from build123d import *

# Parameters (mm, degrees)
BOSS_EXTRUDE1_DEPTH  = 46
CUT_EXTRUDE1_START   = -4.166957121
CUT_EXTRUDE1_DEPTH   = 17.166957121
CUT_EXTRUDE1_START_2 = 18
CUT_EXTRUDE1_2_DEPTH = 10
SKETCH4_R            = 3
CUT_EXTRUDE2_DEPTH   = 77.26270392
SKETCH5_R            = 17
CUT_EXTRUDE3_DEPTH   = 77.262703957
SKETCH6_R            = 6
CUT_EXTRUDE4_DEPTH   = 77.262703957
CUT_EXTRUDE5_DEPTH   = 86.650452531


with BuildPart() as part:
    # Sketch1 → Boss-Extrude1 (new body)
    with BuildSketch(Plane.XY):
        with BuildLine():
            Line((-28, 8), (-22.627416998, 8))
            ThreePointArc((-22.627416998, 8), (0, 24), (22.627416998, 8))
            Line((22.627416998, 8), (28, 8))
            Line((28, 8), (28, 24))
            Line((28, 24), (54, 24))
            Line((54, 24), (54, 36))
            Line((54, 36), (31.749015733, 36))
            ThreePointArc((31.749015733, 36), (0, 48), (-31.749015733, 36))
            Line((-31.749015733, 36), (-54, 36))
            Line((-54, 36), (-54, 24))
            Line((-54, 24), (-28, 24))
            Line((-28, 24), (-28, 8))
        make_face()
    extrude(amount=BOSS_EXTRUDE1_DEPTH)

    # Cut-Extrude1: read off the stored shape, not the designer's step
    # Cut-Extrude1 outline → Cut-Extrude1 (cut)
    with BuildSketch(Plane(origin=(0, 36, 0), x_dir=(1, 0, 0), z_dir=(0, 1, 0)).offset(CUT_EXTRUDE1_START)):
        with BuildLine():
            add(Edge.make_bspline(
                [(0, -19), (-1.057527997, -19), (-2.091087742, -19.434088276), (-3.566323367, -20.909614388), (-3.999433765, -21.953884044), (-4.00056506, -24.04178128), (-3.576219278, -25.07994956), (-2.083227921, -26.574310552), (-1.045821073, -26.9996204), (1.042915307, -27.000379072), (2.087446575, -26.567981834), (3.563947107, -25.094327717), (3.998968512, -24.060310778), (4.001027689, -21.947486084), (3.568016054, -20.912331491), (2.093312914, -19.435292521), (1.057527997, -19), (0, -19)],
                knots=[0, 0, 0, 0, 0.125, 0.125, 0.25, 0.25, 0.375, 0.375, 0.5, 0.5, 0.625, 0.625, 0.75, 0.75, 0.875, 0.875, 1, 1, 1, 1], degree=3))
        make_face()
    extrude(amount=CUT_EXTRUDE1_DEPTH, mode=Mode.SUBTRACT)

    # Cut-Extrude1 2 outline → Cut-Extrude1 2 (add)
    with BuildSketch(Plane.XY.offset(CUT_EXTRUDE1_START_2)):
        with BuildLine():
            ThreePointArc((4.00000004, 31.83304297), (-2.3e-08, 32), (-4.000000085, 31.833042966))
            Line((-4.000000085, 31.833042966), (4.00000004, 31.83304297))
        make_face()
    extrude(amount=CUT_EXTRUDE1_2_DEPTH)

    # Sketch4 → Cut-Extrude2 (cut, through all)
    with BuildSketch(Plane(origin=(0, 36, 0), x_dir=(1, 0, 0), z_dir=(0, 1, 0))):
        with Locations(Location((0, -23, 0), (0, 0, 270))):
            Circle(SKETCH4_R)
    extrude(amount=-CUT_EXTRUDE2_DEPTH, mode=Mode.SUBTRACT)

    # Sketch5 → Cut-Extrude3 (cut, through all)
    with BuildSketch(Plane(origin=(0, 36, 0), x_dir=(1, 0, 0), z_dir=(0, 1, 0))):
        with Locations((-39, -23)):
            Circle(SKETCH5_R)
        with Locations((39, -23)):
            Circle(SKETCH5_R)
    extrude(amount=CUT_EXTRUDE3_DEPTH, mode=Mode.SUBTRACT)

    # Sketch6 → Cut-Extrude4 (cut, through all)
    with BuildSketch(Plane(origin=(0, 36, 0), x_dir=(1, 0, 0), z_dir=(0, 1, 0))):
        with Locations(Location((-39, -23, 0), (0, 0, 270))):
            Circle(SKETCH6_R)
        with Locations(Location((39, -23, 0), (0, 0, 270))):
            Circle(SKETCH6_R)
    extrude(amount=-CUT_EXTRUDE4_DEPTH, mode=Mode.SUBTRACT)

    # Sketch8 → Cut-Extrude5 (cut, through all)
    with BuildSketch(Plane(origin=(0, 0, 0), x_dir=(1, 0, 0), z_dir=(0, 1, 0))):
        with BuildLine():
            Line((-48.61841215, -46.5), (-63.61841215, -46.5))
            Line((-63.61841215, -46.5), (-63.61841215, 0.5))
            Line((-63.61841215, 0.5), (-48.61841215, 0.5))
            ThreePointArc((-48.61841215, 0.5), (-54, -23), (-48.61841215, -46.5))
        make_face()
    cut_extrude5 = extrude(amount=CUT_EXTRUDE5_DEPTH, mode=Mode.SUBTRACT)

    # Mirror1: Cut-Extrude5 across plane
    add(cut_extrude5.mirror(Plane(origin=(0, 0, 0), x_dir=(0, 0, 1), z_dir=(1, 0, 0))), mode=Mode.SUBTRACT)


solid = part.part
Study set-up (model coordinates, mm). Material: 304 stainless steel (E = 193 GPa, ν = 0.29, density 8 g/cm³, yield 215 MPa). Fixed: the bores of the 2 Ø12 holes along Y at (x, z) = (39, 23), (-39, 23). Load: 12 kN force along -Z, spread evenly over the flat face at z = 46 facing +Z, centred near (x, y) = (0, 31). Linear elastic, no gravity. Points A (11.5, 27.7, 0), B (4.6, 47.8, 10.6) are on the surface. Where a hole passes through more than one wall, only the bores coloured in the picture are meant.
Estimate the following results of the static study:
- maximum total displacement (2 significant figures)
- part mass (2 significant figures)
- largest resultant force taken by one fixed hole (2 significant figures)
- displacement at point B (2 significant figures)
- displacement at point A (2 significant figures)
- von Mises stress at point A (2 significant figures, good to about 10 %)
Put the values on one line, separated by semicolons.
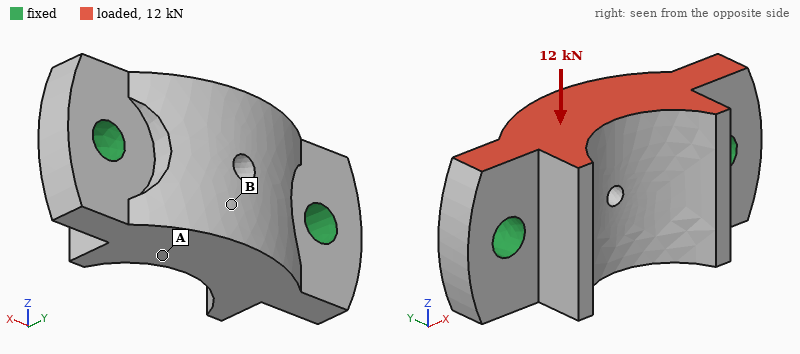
5.5 µm; 750 g; 6.0 kN; 4.4 µm; 3.1 µm; 12 MPa
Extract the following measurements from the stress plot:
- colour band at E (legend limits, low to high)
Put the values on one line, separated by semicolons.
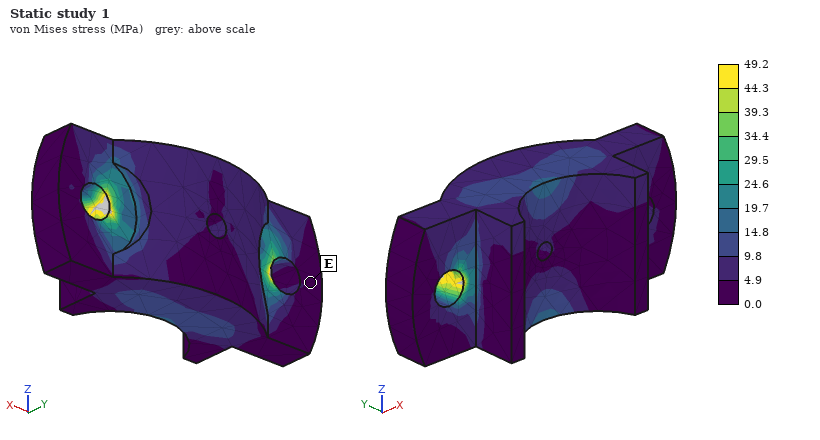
0.0 to 4.9 MPa
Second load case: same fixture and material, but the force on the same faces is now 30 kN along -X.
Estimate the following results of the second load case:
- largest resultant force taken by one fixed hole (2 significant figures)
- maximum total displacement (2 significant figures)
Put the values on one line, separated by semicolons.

17 kN; 14 µm
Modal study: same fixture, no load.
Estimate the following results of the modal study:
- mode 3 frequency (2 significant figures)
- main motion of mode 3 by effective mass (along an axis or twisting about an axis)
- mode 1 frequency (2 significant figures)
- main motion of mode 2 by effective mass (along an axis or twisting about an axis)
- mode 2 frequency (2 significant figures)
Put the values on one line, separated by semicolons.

12 kHz; along Z; 7200 Hz; along Y; 8900 Hz
